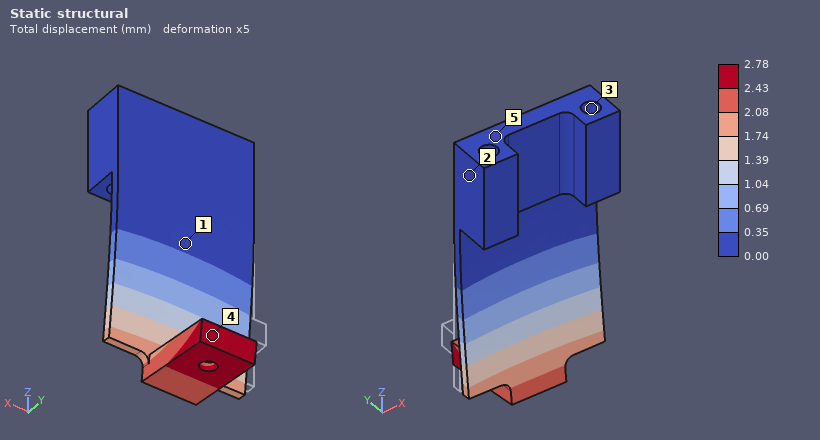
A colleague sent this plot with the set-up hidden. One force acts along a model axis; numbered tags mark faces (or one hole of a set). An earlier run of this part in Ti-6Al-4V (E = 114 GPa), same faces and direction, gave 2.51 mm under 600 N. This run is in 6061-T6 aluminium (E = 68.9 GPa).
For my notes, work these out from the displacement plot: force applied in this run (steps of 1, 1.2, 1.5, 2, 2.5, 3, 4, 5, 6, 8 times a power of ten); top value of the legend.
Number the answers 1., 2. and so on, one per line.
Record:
1. 400 N
2. 2.78 mm
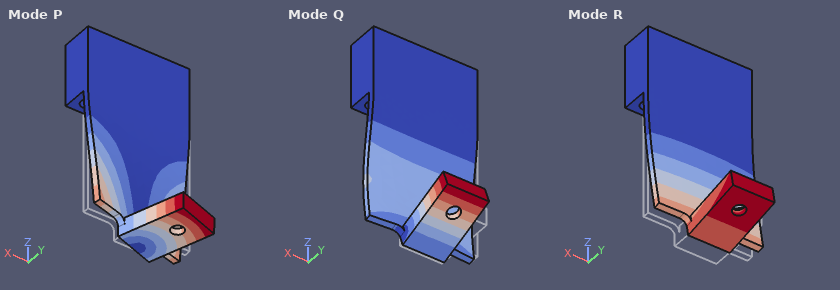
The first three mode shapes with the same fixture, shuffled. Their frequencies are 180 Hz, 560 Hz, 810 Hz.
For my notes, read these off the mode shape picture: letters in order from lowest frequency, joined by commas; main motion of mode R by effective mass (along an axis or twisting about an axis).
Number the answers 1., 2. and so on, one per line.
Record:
1. R, P, Q
2. along Y
